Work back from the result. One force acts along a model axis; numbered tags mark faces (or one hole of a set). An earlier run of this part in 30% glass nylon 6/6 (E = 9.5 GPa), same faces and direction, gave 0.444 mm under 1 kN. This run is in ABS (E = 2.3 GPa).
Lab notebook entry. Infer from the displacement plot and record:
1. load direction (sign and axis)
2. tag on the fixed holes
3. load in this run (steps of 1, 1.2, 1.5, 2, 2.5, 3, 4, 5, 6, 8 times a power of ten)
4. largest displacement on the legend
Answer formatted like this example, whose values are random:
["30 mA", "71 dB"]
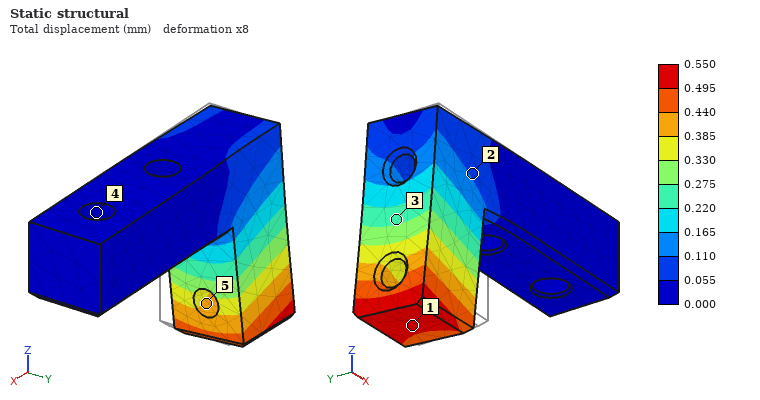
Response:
["+Y", "4", "300 N", "0.550 mm"]
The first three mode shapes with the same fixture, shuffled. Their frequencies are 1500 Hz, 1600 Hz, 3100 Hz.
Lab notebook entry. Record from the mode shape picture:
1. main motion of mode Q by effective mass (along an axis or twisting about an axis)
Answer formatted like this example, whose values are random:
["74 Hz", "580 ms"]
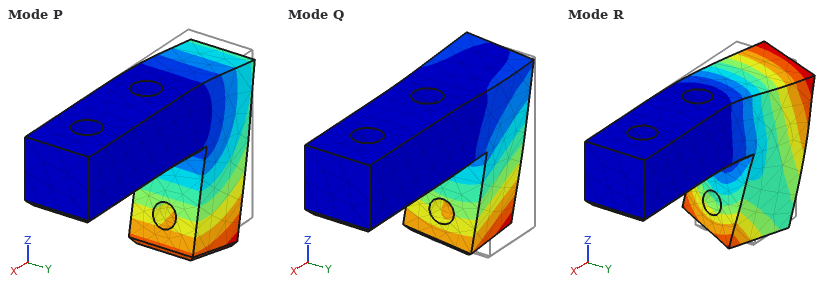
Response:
["along Y"]
